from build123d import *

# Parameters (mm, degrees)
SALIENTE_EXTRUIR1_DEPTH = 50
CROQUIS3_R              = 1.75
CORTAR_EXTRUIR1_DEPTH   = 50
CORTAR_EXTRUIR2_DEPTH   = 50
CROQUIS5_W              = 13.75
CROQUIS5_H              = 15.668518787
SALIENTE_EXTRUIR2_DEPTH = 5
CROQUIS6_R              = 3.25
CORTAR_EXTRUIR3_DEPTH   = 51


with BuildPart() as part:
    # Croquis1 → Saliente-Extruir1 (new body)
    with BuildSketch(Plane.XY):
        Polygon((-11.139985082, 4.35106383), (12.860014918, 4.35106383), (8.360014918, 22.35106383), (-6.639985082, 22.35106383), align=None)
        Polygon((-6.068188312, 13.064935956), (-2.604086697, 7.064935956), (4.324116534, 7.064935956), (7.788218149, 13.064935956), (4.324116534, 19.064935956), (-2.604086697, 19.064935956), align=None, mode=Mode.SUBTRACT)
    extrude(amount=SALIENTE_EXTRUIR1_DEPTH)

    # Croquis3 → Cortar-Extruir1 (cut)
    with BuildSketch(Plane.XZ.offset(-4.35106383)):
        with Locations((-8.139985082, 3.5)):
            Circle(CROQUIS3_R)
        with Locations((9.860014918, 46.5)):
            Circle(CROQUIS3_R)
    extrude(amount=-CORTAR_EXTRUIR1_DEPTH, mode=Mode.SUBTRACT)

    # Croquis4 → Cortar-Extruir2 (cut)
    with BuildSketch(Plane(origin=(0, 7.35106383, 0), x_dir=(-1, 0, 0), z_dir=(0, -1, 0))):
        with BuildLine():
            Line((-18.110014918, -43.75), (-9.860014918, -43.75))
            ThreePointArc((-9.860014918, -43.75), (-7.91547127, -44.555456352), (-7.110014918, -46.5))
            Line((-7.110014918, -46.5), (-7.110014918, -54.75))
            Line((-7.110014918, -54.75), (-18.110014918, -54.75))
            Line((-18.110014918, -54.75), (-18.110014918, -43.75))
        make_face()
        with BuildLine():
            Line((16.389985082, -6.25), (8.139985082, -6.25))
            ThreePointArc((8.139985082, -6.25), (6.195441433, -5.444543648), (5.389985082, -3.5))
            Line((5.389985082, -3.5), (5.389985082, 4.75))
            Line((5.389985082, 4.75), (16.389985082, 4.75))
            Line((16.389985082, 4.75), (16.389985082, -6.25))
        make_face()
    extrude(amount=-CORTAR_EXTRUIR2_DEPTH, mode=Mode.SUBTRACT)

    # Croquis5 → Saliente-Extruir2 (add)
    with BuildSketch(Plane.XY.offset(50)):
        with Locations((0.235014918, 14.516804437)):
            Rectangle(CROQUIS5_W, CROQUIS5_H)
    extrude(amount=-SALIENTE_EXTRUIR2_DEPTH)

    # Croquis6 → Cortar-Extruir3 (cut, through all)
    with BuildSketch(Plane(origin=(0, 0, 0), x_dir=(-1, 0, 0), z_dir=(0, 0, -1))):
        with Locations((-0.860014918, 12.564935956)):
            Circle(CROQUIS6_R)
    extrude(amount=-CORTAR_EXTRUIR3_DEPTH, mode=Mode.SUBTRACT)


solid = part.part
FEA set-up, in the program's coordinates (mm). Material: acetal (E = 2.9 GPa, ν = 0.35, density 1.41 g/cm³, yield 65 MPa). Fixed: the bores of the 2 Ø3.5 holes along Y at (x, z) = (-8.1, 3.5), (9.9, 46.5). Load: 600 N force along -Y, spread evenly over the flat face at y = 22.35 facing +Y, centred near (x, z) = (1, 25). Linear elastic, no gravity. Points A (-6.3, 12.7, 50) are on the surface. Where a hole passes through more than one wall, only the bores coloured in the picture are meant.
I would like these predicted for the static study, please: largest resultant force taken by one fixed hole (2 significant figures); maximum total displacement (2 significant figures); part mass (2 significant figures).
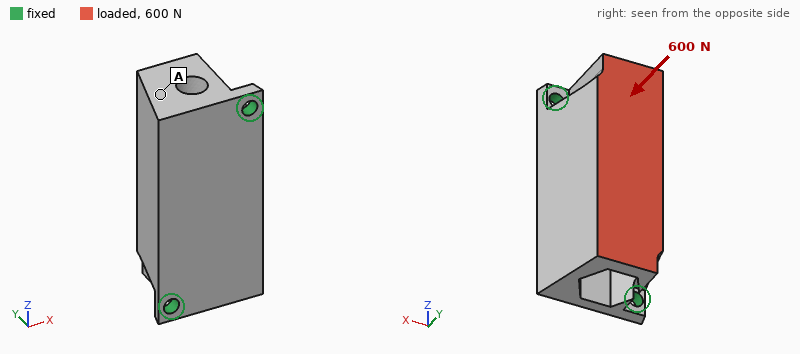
340 N
0.23 mm
16 g
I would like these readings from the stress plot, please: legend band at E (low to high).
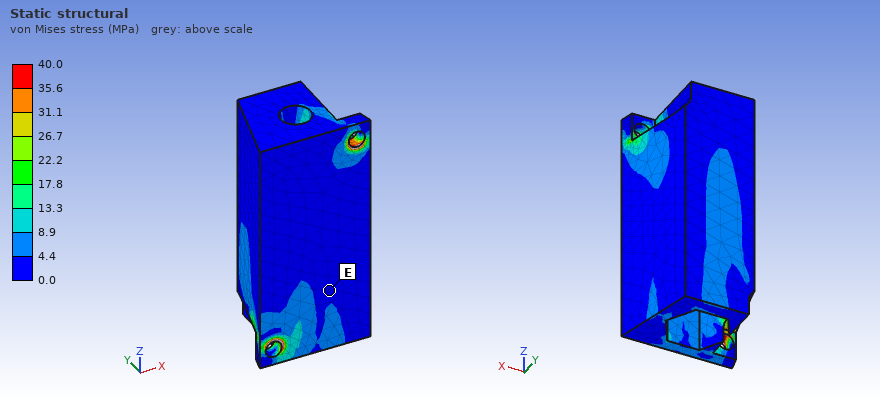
0.0 to 4.4 MPa
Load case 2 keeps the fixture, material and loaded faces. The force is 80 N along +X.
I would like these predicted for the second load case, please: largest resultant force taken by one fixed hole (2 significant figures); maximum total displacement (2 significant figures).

45 N
0.38 mm
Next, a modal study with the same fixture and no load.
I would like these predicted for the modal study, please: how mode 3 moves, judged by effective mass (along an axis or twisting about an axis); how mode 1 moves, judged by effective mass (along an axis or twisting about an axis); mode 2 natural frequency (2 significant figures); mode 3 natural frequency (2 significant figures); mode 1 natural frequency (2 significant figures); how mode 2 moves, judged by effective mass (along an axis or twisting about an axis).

along X
along X
3000 Hz
4100 Hz
900 Hz
along Y
